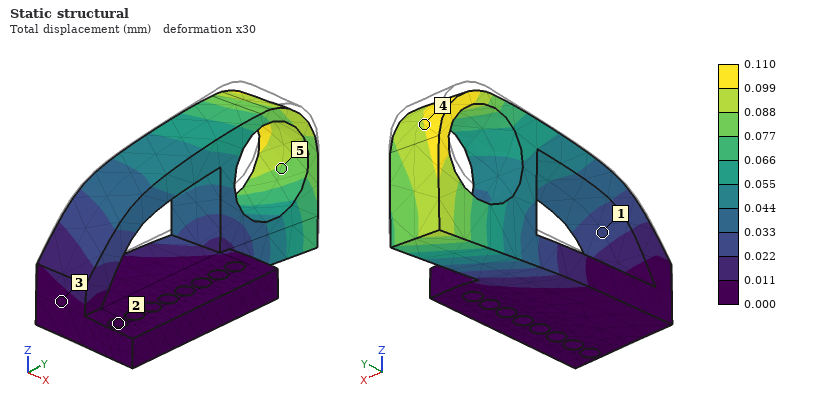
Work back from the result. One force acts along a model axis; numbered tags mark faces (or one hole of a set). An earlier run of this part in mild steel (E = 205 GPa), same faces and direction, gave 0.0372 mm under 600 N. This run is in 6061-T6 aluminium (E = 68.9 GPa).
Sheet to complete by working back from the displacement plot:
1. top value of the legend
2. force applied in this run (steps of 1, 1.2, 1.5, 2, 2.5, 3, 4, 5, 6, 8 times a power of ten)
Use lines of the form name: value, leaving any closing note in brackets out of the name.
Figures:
top value of the legend: 0.110 mm
force applied in this run: 600 N
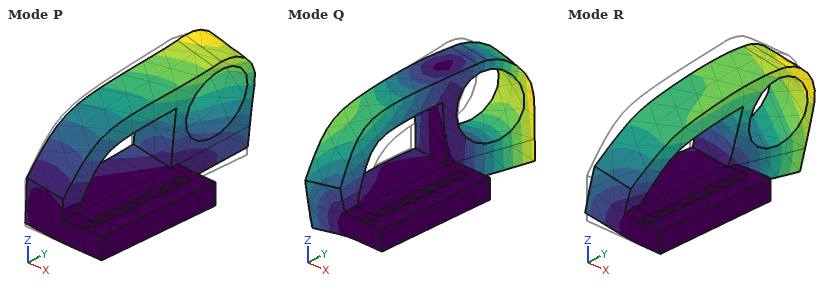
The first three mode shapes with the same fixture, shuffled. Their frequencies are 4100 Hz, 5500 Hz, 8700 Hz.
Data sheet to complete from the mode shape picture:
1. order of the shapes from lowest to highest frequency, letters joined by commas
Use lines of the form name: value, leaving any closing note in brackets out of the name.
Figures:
order of the shapes from lowest to highest frequency, letters joined by commas: P, R, Q
